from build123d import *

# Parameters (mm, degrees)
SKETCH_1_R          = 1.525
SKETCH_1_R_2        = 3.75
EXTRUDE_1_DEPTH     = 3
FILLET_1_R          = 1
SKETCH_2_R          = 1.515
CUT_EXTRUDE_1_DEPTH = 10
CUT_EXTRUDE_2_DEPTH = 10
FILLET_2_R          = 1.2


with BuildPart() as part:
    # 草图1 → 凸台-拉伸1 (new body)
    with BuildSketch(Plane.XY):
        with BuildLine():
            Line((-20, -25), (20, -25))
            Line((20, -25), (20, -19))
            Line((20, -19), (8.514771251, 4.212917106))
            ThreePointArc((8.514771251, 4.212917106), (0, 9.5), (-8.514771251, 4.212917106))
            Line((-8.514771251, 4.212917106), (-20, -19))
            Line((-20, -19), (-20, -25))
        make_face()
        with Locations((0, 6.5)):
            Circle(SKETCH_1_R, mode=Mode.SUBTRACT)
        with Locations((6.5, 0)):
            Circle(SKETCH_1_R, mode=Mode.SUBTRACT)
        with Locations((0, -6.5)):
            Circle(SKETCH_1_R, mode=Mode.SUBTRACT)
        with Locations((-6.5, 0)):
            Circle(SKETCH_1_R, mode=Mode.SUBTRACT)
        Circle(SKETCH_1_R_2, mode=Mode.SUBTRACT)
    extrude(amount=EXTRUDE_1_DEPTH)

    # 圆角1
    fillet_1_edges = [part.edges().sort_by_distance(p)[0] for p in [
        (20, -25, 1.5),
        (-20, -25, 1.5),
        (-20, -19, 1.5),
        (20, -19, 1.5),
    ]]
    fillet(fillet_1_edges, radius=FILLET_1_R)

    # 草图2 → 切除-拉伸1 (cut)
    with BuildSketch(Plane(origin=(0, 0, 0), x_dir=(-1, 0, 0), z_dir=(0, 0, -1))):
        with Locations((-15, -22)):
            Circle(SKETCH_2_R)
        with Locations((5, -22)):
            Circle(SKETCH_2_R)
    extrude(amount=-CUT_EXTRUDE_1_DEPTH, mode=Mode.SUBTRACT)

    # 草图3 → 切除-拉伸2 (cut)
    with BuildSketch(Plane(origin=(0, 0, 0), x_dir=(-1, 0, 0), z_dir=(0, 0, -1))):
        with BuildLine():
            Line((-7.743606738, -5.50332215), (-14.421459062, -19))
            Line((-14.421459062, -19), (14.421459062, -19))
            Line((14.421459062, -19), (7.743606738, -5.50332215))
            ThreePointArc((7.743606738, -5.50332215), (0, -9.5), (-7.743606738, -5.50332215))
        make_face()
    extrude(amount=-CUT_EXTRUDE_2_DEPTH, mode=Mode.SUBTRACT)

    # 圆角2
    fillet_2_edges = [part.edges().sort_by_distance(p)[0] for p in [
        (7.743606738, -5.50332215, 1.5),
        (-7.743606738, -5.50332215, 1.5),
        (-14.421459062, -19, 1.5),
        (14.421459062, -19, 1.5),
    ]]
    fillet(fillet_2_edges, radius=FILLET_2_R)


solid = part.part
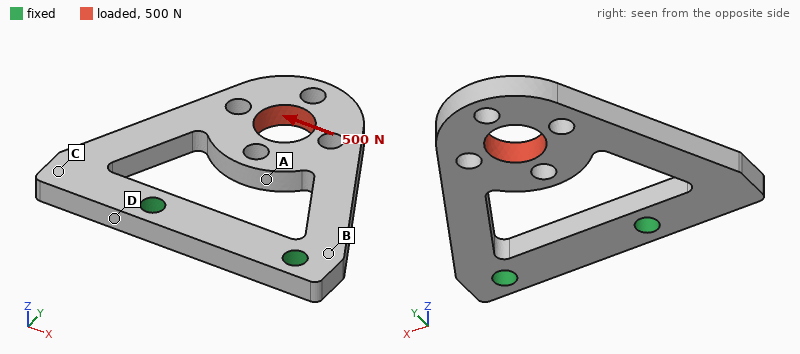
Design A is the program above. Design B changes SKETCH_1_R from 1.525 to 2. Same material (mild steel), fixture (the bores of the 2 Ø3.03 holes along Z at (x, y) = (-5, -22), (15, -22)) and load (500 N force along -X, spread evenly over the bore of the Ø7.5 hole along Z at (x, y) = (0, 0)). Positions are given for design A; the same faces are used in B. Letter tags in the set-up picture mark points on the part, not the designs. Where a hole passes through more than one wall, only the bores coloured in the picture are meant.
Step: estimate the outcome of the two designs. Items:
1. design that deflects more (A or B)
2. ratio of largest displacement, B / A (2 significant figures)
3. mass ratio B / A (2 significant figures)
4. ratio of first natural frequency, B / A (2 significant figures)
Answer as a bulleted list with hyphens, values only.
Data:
- B
- 1.1
- 0.97
- 1.0
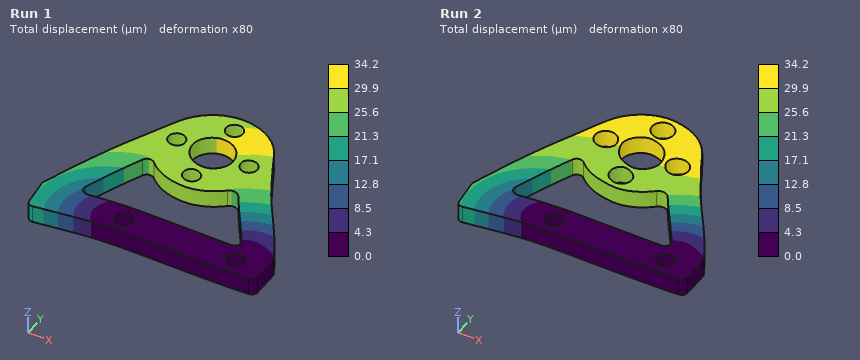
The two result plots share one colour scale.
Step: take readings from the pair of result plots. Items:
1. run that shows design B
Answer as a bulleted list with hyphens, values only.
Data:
- Run 2
